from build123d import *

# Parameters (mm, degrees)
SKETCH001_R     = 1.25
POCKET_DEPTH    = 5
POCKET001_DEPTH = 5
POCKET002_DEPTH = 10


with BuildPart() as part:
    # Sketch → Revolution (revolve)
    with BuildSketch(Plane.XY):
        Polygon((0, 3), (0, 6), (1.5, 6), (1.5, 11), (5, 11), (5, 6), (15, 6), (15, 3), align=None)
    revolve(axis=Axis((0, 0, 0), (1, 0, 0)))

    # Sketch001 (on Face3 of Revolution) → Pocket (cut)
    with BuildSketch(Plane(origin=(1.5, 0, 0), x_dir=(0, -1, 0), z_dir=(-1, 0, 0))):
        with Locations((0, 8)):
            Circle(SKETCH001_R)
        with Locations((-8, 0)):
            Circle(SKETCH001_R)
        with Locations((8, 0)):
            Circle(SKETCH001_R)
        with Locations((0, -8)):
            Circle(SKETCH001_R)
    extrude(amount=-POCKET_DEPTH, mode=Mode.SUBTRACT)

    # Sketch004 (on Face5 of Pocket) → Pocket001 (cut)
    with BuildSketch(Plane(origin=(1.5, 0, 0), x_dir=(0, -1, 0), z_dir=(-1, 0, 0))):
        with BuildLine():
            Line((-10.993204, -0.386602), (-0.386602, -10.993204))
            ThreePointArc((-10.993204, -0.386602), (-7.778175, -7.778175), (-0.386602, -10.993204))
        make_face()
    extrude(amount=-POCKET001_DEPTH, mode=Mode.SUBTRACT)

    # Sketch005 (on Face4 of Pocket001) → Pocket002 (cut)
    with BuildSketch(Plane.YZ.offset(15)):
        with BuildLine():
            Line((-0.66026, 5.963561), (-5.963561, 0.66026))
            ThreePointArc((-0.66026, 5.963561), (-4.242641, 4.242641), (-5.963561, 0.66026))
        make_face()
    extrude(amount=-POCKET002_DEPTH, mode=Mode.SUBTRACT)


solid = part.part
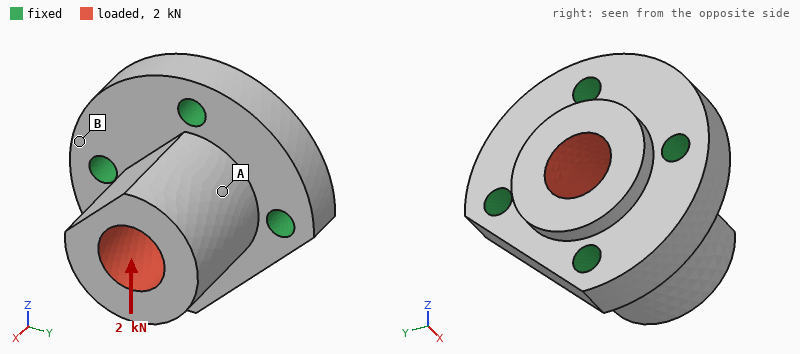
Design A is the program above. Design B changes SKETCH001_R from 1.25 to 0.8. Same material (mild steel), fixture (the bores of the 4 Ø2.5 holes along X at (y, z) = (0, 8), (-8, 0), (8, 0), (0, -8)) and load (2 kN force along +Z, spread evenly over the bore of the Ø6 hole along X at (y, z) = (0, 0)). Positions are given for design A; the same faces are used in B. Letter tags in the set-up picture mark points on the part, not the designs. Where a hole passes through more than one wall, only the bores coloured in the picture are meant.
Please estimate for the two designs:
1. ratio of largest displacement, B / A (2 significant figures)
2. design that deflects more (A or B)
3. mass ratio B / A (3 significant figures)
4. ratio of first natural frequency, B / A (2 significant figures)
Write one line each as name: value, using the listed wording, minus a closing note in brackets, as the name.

ratio of largest displacement, B / A: 1.1
design that deflects more: B
mass ratio B / A: 1.02
ratio of first natural frequency, B / A: 0.94
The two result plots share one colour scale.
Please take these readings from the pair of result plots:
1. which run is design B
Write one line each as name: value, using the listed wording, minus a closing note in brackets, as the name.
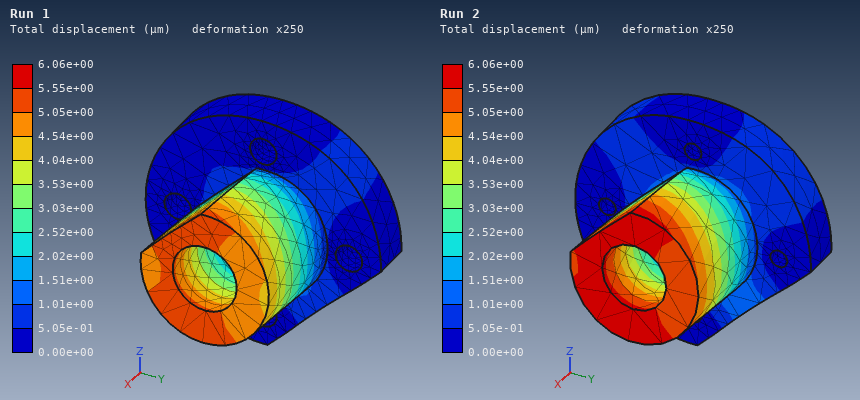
which run is design B: Run 2
